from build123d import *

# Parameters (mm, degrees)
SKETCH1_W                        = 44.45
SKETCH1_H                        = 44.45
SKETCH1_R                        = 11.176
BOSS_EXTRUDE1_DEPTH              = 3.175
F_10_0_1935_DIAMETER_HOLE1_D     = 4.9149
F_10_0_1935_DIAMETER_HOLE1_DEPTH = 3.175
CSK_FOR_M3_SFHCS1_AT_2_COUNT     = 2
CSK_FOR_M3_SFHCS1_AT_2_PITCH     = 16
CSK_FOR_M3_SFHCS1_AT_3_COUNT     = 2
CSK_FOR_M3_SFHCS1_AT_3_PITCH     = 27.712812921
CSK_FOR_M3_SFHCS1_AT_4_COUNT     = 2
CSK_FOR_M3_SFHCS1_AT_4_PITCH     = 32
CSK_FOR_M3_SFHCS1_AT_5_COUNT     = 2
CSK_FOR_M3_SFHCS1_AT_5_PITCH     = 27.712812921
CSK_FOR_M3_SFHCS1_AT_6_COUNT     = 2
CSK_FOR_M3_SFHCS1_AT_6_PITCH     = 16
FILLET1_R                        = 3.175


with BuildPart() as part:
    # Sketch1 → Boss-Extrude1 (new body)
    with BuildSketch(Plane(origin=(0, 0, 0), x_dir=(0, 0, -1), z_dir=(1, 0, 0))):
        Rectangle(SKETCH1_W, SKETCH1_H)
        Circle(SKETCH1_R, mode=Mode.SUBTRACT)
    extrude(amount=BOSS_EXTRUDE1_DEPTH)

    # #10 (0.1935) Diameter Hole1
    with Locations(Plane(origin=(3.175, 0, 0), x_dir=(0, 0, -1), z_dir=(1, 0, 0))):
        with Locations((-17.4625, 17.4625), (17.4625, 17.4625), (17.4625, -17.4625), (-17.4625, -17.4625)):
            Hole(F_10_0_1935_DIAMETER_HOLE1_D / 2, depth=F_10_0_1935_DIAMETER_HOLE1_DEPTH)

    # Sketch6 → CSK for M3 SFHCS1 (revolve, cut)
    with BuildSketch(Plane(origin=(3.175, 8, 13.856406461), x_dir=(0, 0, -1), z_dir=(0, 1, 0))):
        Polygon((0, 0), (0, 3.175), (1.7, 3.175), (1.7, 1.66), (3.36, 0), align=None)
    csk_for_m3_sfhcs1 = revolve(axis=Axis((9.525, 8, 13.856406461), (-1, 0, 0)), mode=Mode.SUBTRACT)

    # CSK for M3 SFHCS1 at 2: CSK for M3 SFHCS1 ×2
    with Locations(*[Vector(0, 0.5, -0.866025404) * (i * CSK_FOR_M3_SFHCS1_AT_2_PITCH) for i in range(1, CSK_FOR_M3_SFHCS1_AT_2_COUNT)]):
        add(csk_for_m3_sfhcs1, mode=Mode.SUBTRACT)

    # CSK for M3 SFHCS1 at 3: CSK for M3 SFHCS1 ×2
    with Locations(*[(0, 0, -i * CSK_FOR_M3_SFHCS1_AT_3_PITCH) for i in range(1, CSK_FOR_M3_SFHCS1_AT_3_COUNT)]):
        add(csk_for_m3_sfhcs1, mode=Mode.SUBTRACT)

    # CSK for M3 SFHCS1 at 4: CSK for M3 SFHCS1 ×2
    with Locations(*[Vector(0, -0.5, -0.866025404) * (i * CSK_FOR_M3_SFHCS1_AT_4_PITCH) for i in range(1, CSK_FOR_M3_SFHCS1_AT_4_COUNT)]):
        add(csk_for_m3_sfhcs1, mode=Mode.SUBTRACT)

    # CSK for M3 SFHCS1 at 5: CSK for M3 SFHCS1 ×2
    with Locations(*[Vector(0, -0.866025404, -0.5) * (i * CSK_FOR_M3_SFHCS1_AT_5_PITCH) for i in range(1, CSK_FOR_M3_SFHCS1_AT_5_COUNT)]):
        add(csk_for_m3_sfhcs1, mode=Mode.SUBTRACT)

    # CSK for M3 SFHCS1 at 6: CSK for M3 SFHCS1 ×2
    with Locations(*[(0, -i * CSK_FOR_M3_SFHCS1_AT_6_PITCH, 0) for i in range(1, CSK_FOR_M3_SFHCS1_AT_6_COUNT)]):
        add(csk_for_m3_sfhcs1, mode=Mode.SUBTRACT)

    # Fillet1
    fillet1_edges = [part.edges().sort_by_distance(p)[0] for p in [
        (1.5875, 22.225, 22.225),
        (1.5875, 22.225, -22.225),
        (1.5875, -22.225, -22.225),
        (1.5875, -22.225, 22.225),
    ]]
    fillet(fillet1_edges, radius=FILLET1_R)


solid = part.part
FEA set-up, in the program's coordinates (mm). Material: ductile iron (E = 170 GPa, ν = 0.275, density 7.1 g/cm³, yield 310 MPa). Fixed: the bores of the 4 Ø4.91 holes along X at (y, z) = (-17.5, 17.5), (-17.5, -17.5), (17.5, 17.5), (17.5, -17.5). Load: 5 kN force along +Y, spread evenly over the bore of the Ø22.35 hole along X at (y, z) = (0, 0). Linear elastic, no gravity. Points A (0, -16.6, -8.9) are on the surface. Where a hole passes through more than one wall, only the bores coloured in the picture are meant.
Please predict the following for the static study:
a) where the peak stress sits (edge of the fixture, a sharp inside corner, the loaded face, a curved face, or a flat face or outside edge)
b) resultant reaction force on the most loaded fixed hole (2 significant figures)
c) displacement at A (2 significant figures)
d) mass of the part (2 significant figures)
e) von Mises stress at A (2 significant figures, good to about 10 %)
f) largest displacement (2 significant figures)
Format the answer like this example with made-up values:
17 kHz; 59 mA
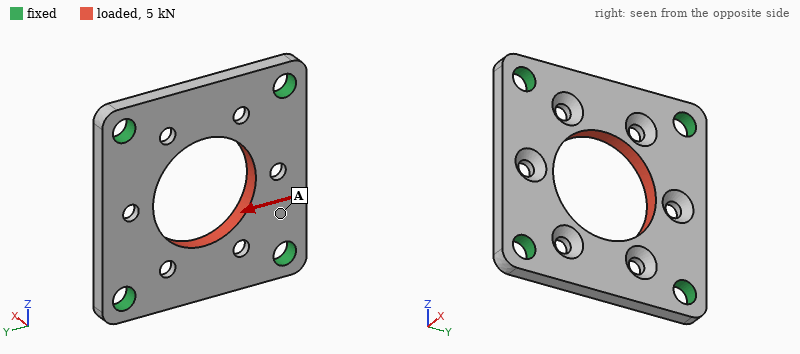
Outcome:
a curved face; 1.3 kN; 3.4 µm; 32 g; 33 MPa; 6.8 µm
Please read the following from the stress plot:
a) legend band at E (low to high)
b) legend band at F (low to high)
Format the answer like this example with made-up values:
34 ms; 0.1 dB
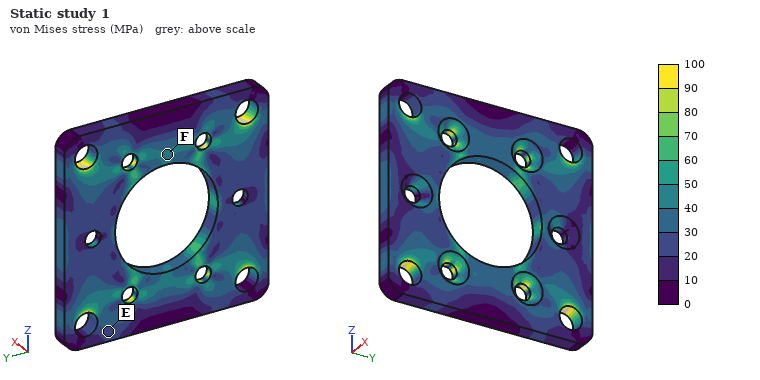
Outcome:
20 to 30 MPa; 40 to 50 MPa
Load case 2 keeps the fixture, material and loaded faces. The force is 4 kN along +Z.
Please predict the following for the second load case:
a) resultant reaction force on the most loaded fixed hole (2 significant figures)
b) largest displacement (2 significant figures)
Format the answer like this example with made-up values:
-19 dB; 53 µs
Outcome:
1.0 kN; 5.7 µm
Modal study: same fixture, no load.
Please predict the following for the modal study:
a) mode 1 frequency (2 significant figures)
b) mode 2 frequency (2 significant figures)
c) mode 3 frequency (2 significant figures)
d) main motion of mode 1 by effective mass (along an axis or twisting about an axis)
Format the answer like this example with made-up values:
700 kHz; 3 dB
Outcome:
13 kHz; 15 kHz; 16 kHz; along X
